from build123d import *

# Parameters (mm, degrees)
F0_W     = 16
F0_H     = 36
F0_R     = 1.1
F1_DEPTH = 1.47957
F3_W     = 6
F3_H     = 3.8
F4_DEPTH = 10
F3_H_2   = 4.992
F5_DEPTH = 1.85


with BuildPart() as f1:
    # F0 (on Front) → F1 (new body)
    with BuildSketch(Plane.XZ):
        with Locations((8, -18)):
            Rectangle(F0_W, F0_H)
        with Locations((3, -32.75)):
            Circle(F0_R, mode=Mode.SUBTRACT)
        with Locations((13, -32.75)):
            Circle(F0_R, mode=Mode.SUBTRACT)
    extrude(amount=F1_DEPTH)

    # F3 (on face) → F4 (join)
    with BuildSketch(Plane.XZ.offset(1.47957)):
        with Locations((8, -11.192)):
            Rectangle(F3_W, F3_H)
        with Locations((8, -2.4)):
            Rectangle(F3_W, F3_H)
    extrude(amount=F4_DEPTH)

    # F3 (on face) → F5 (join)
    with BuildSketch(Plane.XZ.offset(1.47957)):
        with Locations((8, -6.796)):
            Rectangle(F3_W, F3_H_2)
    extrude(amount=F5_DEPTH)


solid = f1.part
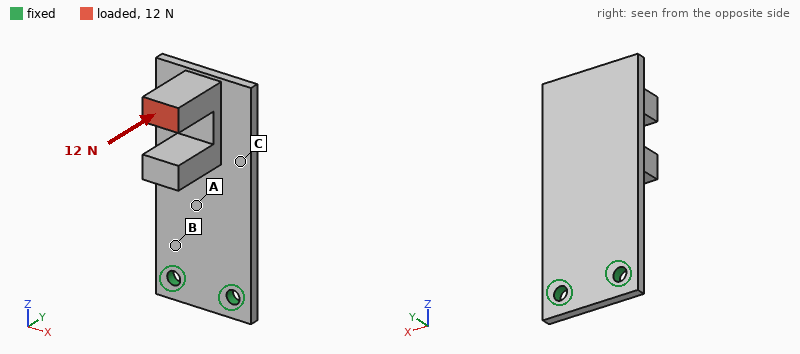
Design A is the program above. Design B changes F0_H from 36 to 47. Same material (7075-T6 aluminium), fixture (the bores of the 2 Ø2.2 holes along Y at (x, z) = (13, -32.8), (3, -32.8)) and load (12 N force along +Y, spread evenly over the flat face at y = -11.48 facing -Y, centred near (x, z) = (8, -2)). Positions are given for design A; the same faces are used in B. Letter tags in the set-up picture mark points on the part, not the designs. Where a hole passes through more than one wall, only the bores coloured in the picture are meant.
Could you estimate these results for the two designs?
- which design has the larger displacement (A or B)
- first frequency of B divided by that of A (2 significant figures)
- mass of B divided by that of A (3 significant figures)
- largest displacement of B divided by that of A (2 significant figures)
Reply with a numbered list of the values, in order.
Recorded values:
1. B
2. 0.87
3. 1.19
4. 1.1
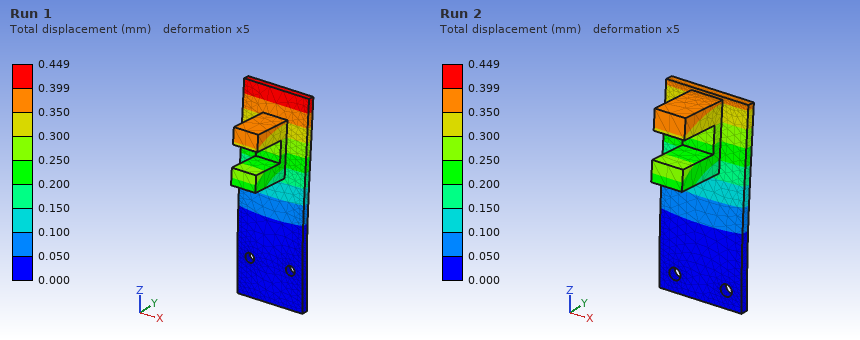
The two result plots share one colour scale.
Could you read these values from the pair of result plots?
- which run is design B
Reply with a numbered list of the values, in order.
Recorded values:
1. Run 1
